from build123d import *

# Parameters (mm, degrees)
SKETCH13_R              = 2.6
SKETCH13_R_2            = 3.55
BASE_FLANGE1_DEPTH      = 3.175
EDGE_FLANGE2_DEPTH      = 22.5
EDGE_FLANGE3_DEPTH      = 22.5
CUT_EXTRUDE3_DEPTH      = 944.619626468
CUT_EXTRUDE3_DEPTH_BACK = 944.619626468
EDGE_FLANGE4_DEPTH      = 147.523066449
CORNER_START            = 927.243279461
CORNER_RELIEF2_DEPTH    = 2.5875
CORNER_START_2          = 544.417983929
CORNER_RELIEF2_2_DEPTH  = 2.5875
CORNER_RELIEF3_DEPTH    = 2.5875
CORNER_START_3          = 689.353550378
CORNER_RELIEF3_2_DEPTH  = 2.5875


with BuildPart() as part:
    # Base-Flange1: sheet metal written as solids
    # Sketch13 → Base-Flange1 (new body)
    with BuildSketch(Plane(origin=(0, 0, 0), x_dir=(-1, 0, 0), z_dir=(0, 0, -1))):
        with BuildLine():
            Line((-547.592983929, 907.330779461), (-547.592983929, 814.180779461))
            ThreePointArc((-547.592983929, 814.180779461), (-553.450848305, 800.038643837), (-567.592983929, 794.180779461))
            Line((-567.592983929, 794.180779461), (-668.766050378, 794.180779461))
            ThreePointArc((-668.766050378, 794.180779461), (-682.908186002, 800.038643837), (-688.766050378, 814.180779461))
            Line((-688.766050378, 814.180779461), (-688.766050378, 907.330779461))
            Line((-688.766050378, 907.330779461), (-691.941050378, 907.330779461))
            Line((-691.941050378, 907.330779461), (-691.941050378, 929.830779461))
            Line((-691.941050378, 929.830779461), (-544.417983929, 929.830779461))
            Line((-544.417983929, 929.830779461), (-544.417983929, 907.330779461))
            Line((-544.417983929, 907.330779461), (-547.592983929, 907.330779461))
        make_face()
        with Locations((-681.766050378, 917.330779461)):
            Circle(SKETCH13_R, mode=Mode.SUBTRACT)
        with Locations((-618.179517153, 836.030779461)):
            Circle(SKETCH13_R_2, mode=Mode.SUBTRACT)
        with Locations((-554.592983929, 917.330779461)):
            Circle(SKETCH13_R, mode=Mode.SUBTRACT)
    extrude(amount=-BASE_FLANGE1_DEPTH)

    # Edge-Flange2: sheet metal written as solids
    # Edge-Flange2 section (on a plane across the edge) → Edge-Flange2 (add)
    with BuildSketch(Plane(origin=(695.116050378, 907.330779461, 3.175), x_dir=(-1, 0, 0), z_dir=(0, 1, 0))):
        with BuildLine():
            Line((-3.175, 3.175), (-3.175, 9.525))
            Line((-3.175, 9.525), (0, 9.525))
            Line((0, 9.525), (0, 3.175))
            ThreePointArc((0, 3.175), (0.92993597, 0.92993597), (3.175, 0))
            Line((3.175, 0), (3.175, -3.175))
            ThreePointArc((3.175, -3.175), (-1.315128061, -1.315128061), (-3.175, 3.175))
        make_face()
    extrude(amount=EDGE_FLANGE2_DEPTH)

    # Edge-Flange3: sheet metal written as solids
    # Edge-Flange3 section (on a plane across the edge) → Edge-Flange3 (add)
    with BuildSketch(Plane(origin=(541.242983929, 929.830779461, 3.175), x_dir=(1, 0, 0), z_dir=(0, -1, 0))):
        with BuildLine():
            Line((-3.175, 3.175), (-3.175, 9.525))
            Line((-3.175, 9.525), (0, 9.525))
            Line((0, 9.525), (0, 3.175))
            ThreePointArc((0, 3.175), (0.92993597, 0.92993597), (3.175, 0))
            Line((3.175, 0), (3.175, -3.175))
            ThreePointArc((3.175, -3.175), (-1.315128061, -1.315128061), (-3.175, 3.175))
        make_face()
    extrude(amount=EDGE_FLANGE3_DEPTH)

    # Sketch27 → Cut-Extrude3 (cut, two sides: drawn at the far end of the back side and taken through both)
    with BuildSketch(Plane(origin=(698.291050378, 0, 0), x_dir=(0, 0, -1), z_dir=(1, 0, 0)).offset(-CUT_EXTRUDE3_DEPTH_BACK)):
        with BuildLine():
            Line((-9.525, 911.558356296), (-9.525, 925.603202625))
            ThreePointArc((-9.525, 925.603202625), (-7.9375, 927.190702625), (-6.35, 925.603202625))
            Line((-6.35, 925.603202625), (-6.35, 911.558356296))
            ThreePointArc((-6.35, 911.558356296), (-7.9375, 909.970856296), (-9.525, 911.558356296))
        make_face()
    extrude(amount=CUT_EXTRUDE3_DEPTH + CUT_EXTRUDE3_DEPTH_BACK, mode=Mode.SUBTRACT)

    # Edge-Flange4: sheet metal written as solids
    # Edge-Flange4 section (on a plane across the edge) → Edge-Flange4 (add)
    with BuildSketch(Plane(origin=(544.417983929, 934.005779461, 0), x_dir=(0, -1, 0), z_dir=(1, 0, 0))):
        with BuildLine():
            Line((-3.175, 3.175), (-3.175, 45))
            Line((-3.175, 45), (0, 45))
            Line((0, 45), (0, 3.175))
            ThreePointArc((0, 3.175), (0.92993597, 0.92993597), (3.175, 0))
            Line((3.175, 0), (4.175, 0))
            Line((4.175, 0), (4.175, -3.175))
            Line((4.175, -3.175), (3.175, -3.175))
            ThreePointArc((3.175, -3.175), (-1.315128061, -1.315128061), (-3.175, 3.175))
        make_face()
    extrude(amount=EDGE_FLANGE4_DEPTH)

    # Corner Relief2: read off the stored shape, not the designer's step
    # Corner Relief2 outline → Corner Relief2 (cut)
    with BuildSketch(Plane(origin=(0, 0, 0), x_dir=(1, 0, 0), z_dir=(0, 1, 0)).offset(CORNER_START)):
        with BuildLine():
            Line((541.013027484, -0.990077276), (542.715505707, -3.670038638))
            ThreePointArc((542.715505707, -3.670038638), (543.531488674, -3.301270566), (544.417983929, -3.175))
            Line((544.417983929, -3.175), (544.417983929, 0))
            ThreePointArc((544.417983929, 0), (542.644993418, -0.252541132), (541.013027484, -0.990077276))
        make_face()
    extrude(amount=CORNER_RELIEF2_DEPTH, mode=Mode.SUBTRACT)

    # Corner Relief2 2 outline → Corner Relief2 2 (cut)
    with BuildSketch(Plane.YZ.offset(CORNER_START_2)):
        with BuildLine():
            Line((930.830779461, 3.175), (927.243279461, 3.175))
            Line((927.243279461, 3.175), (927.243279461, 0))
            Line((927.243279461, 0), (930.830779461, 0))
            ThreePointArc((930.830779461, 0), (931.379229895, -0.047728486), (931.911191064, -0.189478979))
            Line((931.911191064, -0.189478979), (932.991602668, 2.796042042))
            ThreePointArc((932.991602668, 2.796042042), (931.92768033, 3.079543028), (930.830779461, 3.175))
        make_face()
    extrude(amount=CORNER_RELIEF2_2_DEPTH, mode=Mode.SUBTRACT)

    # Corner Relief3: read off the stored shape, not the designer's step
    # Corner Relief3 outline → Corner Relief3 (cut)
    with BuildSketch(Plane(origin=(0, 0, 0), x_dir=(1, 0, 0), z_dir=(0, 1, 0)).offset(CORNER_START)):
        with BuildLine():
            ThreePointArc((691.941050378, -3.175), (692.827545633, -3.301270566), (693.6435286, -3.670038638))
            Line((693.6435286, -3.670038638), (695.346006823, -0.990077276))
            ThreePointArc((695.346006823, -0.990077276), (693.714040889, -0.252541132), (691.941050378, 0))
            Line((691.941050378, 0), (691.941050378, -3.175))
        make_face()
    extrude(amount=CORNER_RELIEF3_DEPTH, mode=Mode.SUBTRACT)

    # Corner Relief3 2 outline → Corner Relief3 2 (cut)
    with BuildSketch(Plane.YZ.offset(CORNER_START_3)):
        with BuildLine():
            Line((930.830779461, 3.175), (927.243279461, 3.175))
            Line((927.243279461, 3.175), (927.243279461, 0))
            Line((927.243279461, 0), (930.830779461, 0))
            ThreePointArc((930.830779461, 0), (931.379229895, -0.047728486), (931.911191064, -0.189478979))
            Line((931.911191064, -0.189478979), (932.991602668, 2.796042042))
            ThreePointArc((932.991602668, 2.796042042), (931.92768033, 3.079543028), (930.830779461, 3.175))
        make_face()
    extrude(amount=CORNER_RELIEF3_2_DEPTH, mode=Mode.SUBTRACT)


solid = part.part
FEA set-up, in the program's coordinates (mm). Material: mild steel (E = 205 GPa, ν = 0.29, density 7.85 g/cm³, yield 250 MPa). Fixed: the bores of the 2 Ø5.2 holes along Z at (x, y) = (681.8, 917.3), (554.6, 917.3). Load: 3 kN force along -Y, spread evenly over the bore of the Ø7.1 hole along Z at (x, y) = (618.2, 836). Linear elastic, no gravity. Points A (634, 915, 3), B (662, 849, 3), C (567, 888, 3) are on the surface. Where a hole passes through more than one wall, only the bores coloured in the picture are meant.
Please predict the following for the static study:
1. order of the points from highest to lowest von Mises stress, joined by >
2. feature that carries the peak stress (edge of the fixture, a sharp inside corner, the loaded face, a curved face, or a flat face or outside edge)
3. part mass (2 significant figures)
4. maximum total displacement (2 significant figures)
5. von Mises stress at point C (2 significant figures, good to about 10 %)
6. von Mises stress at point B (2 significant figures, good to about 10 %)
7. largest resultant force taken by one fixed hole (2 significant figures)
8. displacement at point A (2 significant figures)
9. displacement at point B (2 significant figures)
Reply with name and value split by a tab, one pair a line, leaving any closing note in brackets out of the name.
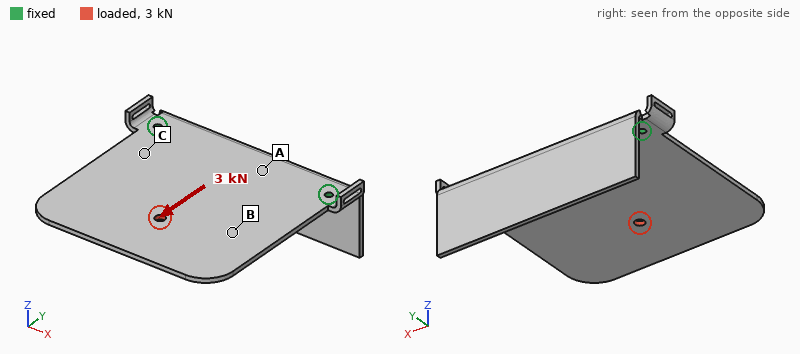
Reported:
order of the points from highest to lowest von Mises stress, joined by >	C > B > A
feature that carries the peak stress	the loaded face
part mass	670 g
maximum total displacement	9.0 µm
von Mises stress at point C	12 MPa
von Mises stress at point B	6.2 MPa
largest resultant force taken by one fixed hole	1.5 kN
displacement at point A	4.7 µm
displacement at point B	4.4 µm
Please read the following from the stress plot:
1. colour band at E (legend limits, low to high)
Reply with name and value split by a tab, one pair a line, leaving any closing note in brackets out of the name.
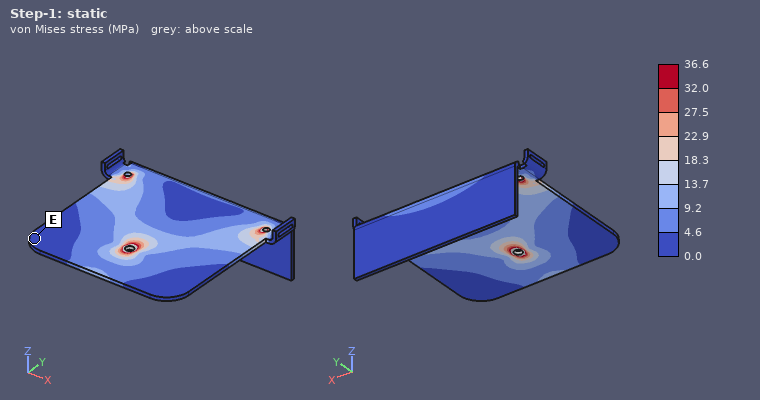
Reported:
colour band at E	0.0 to 4.6 MPa
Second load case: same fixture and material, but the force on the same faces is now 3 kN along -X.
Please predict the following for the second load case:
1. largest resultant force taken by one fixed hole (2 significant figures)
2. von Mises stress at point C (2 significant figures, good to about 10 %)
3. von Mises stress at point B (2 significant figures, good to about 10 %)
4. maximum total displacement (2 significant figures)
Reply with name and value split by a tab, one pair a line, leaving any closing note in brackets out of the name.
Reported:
largest resultant force taken by one fixed hole	2.4 kN
von Mises stress at point C	17 MPa
von Mises stress at point B	9.4 MPa
maximum total displacement	17 µm
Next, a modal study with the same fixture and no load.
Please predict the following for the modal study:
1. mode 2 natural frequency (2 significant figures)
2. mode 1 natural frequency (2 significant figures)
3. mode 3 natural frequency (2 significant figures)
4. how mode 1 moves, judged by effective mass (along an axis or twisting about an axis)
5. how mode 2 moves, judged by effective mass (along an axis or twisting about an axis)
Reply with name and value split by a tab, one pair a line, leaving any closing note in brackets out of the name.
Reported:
mode 2 natural frequency	410 Hz
mode 1 natural frequency	150 Hz
mode 3 natural frequency	660 Hz
how mode 1 moves, judged by effective mass	along Z
how mode 2 moves, judged by effective mass	twisting about Y
